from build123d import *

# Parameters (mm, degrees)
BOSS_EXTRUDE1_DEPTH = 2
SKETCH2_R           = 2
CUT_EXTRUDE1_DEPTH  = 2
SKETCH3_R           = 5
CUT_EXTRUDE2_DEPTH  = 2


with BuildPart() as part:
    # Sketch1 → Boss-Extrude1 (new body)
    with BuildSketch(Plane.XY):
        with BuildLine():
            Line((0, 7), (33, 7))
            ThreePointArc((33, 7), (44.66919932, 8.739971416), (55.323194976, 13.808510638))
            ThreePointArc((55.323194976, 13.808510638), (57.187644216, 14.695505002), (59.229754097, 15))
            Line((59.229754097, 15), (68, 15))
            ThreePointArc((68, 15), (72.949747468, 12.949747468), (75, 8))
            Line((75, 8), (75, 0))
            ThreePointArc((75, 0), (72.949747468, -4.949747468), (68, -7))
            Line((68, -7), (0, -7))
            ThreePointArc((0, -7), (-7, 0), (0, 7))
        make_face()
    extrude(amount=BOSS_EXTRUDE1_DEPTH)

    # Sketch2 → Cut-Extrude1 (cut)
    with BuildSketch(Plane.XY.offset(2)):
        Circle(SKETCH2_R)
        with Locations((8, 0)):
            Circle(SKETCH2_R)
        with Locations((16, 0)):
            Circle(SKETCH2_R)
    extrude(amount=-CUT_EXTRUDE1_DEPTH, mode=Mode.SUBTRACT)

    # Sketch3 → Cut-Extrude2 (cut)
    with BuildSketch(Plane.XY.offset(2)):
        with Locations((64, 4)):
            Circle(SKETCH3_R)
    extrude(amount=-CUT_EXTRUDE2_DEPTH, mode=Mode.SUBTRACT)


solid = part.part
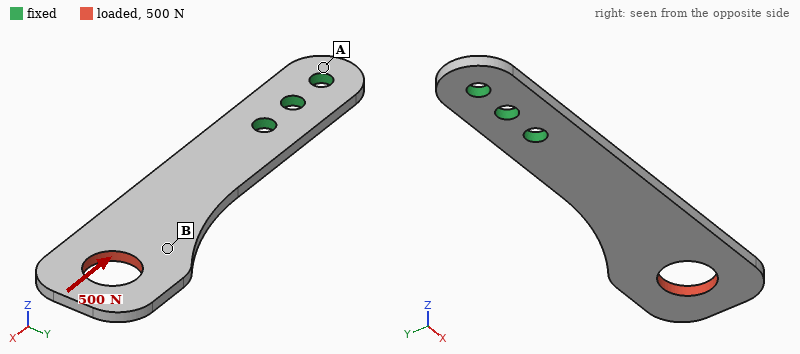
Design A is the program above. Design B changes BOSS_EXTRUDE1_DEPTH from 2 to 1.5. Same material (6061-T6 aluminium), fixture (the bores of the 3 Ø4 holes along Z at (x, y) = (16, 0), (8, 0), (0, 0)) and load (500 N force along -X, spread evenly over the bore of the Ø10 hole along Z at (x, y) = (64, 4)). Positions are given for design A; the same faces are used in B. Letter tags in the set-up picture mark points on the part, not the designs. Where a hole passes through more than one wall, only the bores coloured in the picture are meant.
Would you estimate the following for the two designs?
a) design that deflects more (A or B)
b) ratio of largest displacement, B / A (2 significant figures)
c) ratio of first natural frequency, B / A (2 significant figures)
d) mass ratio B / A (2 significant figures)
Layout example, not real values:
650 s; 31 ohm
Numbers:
B; 1.3; 0.75; 0.75
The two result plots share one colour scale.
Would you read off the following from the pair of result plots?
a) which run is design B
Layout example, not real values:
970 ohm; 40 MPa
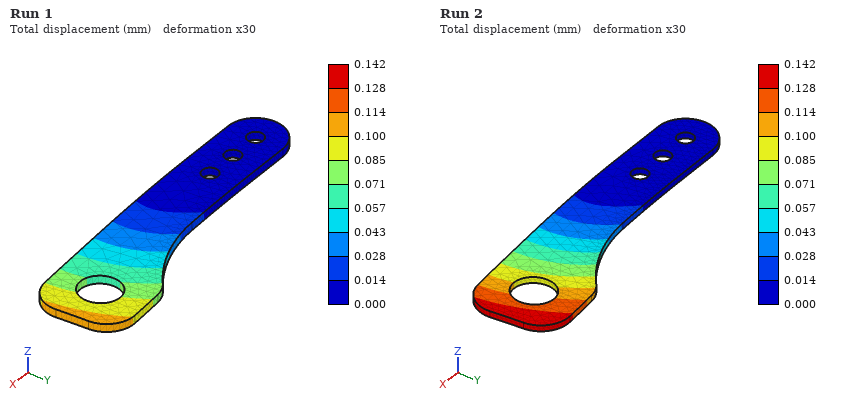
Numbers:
Run 2
